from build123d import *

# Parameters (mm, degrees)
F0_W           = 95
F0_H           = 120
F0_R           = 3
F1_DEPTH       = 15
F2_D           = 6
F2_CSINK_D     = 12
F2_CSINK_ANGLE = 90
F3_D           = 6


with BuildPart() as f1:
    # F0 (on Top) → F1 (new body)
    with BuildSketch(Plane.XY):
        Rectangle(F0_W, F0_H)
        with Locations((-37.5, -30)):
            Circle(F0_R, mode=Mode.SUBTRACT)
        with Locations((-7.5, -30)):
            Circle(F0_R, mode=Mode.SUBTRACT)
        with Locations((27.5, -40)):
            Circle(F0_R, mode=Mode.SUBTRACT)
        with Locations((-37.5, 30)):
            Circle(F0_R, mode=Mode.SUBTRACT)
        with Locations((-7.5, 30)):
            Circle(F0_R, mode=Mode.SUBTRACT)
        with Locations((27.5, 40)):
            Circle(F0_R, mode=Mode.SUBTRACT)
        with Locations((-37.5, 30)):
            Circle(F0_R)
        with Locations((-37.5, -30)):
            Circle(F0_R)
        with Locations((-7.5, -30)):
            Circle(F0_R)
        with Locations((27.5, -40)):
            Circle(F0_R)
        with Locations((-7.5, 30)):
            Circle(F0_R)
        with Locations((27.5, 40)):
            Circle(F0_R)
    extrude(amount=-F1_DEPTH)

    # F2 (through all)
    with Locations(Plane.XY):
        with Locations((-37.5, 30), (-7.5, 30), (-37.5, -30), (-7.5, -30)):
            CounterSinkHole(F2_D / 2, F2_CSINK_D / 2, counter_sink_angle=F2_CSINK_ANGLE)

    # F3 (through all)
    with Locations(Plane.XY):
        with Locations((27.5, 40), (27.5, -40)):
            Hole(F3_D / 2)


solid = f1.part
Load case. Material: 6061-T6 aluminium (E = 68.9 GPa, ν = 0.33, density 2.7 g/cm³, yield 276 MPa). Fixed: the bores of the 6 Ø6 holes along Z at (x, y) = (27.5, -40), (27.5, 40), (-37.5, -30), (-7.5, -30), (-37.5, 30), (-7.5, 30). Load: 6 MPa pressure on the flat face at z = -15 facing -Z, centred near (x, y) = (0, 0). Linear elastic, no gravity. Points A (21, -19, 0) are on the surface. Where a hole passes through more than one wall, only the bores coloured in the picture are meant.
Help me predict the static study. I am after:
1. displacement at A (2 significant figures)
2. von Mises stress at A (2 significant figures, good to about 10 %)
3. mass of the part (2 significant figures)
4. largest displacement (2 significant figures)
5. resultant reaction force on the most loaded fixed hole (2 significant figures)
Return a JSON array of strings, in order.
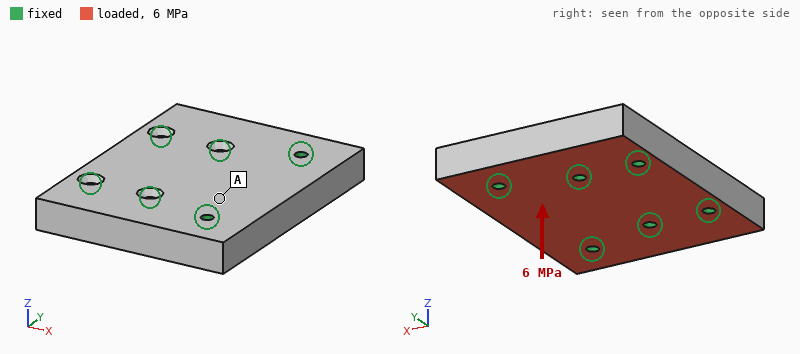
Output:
["29 µm", "17 MPa", "450 g", "65 µm", "14 kN"]
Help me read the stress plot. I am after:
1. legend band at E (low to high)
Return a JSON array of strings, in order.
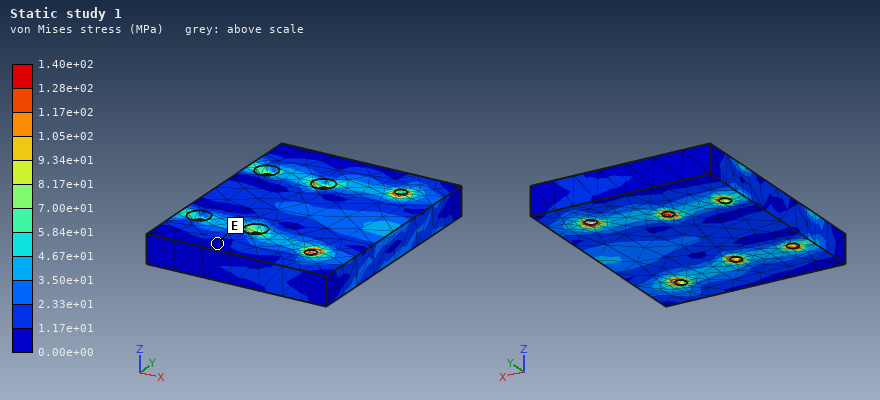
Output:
["0.00e+00 to 1.17e+01 MPa"]
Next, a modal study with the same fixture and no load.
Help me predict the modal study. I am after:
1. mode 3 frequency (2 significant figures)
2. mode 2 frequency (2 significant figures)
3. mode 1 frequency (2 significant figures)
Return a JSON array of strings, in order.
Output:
["11 kHz", "11 kHz", "9100 Hz"]
